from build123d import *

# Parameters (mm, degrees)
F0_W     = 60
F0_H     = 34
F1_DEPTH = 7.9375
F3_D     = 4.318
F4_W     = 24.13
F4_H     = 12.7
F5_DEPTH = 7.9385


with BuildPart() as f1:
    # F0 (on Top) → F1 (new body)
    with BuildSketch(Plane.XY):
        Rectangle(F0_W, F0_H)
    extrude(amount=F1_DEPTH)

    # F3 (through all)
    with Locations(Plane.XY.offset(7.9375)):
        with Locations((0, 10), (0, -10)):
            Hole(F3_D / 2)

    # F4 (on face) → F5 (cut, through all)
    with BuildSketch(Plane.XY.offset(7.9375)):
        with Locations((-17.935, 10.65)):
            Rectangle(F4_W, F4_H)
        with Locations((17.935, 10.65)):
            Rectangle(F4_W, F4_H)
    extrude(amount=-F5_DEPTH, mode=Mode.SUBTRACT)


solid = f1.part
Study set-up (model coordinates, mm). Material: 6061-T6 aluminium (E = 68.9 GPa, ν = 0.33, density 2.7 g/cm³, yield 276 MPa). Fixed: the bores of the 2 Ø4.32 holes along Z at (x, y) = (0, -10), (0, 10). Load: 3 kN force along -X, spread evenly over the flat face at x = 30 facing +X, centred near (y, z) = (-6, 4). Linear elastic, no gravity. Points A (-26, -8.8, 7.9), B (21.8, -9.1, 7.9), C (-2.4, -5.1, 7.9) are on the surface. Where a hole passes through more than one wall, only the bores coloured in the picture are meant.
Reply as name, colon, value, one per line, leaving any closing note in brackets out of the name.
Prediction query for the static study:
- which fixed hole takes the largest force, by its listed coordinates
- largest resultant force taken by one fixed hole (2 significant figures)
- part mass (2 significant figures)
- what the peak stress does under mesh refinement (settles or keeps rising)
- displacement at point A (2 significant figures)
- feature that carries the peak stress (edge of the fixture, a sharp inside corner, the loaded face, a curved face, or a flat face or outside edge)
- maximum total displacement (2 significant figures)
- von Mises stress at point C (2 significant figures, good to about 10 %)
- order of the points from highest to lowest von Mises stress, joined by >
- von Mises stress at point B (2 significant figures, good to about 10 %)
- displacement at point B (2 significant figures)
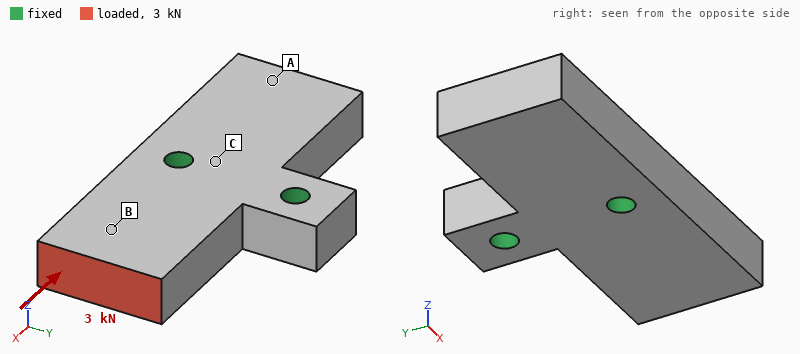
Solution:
which fixed hole takes the largest force, by its listed coordinates: (0, -10)
largest resultant force taken by one fixed hole: 2.4 kN
part mass: 30 g
what the peak stress does under mesh refinement: keeps rising
displacement at point A: 1.4 µm
feature that carries the peak stress: edge of the fixture
maximum total displacement: 9.0 µm
von Mises stress at point C: 11 MPa
order of the points from highest to lowest von Mises stress, joined by >: B > C > A
von Mises stress at point B: 18 MPa
displacement at point B: 6.1 µm
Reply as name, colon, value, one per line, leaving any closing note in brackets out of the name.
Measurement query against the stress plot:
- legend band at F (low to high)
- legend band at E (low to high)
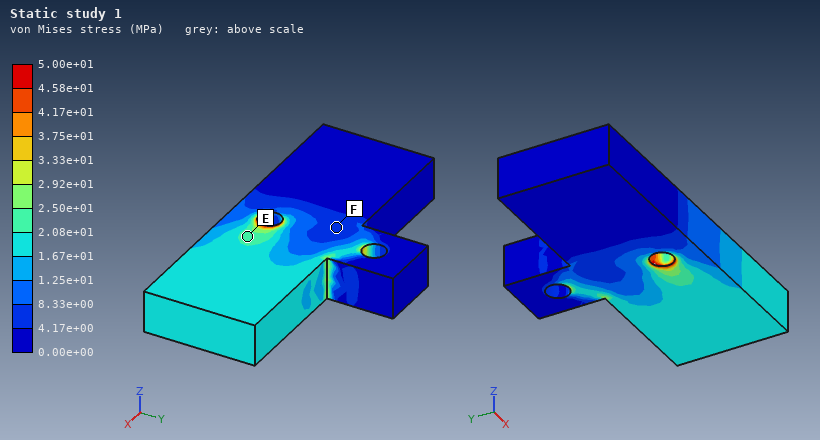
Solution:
legend band at F: 4.17e+00 to 8.33e+00 MPa
legend band at E: 2.08e+01 to 2.50e+01 MPa
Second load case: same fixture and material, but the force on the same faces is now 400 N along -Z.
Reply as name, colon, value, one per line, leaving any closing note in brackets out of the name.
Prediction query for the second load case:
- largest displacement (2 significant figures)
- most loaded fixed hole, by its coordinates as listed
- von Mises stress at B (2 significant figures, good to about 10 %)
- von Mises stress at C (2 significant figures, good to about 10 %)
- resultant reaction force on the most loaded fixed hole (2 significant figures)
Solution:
largest displacement: 64 µm
most loaded fixed hole, by its coordinates as listed: (0, -10)
von Mises stress at B: 15 MPa
von Mises stress at C: 13 MPa
resultant reaction force on the most loaded fixed hole: 340 N
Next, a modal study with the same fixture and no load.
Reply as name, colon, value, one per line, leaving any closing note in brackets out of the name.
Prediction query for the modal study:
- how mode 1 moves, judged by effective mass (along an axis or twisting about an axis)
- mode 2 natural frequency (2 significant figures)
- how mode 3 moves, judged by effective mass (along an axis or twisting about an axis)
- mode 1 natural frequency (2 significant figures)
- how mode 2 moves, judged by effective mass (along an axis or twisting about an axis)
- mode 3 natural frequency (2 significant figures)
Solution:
how mode 1 moves, judged by effective mass: twisting about Y
mode 2 natural frequency: 7400 Hz
how mode 3 moves, judged by effective mass: twisting about Z
mode 1 natural frequency: 6300 Hz
how mode 2 moves, judged by effective mass: along Z
mode 3 natural frequency: 12 kHz
